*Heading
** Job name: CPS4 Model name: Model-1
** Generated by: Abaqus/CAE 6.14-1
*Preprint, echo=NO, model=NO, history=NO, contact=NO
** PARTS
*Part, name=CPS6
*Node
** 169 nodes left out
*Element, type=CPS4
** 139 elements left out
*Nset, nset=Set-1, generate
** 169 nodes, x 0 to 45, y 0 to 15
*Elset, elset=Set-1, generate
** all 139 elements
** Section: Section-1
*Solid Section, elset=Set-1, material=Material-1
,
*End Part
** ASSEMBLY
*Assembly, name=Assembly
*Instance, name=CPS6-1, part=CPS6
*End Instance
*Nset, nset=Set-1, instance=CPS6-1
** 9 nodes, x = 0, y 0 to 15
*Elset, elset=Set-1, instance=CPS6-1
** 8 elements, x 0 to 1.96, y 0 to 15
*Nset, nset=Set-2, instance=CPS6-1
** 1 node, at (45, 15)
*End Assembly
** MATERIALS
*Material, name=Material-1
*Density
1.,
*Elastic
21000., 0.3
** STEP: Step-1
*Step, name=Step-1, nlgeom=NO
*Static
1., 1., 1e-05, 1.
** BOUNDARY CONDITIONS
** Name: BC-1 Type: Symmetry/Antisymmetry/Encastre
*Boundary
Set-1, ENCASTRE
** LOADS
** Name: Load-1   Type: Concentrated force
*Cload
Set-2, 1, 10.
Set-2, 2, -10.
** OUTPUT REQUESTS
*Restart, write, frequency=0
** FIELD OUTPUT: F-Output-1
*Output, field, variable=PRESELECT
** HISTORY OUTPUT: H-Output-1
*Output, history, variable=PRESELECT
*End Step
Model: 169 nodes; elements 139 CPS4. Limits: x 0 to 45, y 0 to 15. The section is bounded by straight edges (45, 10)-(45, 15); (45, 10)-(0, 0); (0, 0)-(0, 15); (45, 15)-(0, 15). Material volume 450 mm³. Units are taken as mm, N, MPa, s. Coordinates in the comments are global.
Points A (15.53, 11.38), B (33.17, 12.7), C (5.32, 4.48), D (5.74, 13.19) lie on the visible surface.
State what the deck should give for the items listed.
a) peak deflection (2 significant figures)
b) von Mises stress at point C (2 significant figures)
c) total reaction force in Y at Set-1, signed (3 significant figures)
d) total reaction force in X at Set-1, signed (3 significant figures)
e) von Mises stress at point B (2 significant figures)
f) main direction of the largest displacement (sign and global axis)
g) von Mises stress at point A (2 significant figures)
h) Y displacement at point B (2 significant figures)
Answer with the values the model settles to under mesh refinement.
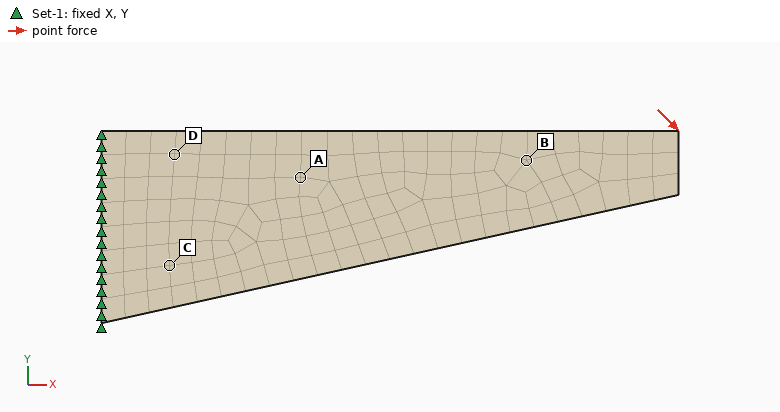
0.15 mm
7.5 MPa
10.0 N
-10.0 N
7.8 MPa
-Y
6.7 MPa
-0.070 mm
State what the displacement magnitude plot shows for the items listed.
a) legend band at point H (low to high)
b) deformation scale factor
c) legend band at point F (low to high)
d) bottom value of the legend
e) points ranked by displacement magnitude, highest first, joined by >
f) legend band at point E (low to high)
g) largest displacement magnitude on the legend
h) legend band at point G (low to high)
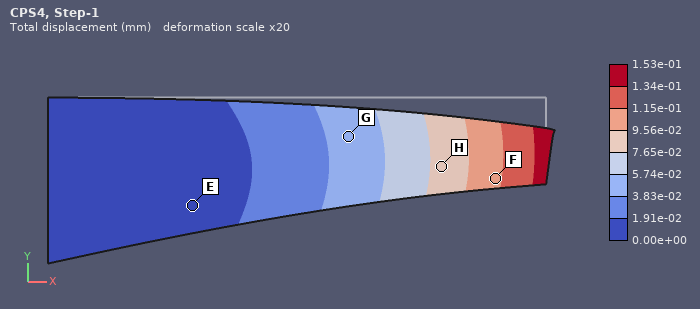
7.65e-02 to 9.56e-02 mm
20
9.56e-02 to 1.15e-01 mm
0.00e+00 mm
F > H > G > E
0.00e+00 to 1.91e-02 mm
1.53e-01 mm
3.83e-02 to 5.74e-02 mm
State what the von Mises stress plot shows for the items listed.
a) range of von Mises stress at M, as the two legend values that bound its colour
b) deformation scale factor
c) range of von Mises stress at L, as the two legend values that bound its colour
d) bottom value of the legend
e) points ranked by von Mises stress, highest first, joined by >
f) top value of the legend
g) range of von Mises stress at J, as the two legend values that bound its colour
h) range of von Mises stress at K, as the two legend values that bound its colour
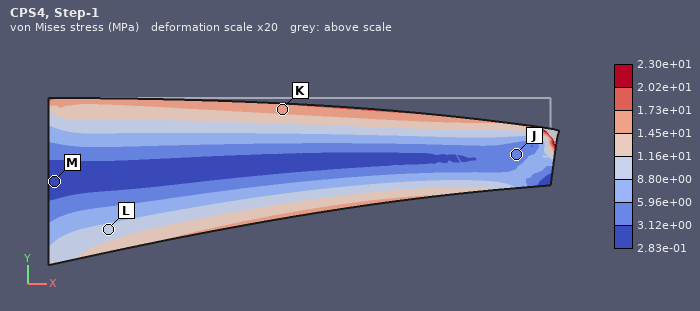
2.83e-01 to 3.12e+00 MPa
20
8.80e+00 to 1.16e+01 MPa
2.83e-01 MPa
K > L > J > M
2.30e+01 MPa
3.12e+00 to 5.96e+00 MPa
1.45e+01 to 1.73e+01 MPa
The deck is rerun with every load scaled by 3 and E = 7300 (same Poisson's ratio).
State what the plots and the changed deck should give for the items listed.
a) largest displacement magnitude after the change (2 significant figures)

1.3 mm
